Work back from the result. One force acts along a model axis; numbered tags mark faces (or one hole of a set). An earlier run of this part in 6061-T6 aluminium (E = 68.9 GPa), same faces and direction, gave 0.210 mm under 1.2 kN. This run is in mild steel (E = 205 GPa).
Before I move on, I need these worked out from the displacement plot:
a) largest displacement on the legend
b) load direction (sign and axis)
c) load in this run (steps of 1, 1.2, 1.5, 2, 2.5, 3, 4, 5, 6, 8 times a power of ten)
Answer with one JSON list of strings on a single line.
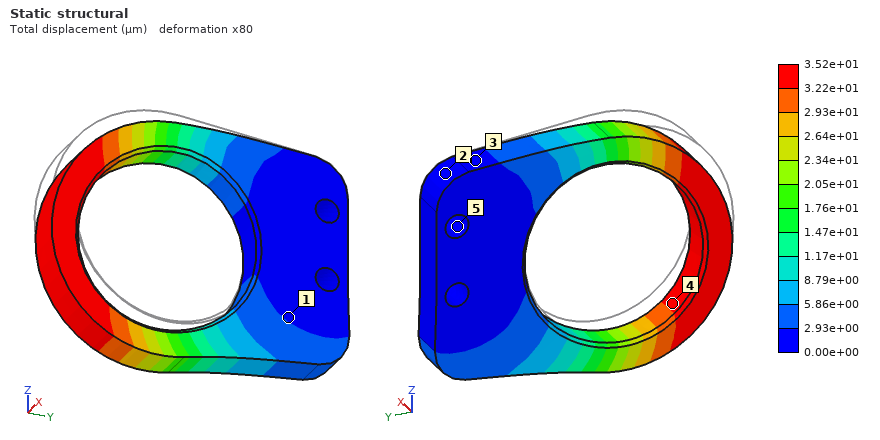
["3.52e+01 µm", "-Z", "600 N"]
